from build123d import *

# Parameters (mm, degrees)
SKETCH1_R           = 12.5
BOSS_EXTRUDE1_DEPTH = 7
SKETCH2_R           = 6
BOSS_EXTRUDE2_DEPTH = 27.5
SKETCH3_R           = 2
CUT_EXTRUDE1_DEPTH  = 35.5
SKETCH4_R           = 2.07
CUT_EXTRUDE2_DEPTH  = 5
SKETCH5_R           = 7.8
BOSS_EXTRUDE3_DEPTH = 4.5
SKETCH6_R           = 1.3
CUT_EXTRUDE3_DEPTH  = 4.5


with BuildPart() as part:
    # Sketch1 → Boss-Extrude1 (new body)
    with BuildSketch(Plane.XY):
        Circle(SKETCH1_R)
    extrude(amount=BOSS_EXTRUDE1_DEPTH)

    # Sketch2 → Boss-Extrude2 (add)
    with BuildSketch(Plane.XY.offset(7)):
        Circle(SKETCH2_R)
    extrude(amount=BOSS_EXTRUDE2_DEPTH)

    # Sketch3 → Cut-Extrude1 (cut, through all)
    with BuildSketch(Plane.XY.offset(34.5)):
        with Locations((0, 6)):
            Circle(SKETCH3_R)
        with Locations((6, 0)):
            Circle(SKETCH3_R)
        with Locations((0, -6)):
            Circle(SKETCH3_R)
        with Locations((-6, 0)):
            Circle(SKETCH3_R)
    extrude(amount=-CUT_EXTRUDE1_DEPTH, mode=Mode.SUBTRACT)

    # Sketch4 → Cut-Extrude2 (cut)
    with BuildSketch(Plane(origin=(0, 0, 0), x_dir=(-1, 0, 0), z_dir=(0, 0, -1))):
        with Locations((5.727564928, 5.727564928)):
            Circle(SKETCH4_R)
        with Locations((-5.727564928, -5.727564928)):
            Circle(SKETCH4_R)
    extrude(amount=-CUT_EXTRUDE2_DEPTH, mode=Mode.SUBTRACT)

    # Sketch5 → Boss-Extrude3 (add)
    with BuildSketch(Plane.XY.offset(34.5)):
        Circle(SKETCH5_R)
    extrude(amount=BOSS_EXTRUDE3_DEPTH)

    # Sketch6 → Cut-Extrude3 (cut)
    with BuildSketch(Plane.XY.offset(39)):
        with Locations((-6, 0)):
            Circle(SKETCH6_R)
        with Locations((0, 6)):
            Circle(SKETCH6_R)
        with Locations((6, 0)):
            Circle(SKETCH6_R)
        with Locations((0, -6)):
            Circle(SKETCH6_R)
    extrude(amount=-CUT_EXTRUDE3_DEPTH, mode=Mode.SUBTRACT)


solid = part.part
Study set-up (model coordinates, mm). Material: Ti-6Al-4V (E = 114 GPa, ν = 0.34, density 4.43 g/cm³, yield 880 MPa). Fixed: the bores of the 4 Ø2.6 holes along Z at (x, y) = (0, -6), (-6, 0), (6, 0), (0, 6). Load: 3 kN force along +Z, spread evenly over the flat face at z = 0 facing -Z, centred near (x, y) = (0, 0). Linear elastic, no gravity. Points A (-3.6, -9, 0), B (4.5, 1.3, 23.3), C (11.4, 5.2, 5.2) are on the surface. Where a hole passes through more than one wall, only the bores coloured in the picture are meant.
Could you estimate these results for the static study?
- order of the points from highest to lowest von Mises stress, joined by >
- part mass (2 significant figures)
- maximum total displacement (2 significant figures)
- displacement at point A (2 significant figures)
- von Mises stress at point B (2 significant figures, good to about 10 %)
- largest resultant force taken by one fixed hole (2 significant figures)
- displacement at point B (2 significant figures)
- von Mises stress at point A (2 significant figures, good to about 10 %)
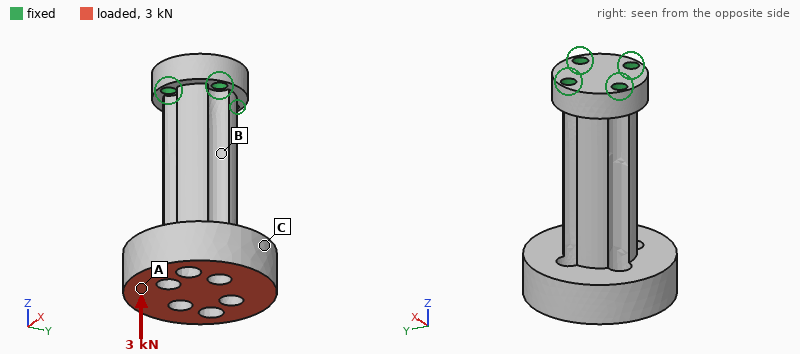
B > A > C
27 g
14 µm
13 µm
34 MPa
790 N
4.5 µm
19 MPa
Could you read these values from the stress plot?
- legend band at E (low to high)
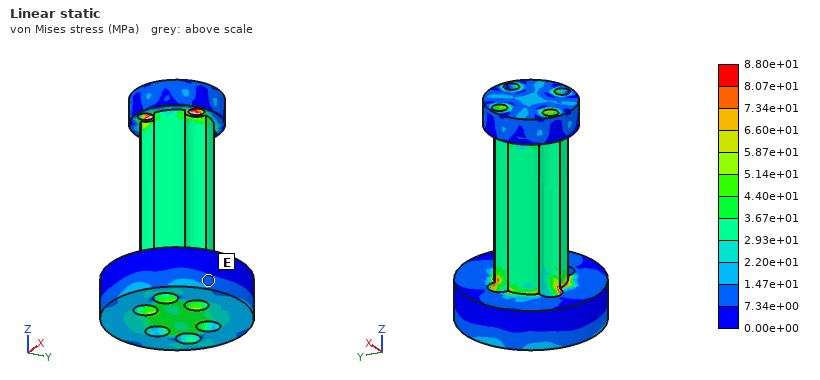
7.34e+00 to 1.47e+01 MPa
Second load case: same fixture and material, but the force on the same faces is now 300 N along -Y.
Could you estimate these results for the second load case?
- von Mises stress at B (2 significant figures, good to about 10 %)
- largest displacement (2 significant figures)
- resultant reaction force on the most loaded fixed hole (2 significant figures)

16 MPa
73 µm
850 N
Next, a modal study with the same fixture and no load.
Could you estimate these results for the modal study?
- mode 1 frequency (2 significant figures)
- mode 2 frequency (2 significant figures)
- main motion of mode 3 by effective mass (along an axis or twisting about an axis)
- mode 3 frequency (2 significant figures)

3100 Hz
3100 Hz
twisting about Z
5400 Hz
